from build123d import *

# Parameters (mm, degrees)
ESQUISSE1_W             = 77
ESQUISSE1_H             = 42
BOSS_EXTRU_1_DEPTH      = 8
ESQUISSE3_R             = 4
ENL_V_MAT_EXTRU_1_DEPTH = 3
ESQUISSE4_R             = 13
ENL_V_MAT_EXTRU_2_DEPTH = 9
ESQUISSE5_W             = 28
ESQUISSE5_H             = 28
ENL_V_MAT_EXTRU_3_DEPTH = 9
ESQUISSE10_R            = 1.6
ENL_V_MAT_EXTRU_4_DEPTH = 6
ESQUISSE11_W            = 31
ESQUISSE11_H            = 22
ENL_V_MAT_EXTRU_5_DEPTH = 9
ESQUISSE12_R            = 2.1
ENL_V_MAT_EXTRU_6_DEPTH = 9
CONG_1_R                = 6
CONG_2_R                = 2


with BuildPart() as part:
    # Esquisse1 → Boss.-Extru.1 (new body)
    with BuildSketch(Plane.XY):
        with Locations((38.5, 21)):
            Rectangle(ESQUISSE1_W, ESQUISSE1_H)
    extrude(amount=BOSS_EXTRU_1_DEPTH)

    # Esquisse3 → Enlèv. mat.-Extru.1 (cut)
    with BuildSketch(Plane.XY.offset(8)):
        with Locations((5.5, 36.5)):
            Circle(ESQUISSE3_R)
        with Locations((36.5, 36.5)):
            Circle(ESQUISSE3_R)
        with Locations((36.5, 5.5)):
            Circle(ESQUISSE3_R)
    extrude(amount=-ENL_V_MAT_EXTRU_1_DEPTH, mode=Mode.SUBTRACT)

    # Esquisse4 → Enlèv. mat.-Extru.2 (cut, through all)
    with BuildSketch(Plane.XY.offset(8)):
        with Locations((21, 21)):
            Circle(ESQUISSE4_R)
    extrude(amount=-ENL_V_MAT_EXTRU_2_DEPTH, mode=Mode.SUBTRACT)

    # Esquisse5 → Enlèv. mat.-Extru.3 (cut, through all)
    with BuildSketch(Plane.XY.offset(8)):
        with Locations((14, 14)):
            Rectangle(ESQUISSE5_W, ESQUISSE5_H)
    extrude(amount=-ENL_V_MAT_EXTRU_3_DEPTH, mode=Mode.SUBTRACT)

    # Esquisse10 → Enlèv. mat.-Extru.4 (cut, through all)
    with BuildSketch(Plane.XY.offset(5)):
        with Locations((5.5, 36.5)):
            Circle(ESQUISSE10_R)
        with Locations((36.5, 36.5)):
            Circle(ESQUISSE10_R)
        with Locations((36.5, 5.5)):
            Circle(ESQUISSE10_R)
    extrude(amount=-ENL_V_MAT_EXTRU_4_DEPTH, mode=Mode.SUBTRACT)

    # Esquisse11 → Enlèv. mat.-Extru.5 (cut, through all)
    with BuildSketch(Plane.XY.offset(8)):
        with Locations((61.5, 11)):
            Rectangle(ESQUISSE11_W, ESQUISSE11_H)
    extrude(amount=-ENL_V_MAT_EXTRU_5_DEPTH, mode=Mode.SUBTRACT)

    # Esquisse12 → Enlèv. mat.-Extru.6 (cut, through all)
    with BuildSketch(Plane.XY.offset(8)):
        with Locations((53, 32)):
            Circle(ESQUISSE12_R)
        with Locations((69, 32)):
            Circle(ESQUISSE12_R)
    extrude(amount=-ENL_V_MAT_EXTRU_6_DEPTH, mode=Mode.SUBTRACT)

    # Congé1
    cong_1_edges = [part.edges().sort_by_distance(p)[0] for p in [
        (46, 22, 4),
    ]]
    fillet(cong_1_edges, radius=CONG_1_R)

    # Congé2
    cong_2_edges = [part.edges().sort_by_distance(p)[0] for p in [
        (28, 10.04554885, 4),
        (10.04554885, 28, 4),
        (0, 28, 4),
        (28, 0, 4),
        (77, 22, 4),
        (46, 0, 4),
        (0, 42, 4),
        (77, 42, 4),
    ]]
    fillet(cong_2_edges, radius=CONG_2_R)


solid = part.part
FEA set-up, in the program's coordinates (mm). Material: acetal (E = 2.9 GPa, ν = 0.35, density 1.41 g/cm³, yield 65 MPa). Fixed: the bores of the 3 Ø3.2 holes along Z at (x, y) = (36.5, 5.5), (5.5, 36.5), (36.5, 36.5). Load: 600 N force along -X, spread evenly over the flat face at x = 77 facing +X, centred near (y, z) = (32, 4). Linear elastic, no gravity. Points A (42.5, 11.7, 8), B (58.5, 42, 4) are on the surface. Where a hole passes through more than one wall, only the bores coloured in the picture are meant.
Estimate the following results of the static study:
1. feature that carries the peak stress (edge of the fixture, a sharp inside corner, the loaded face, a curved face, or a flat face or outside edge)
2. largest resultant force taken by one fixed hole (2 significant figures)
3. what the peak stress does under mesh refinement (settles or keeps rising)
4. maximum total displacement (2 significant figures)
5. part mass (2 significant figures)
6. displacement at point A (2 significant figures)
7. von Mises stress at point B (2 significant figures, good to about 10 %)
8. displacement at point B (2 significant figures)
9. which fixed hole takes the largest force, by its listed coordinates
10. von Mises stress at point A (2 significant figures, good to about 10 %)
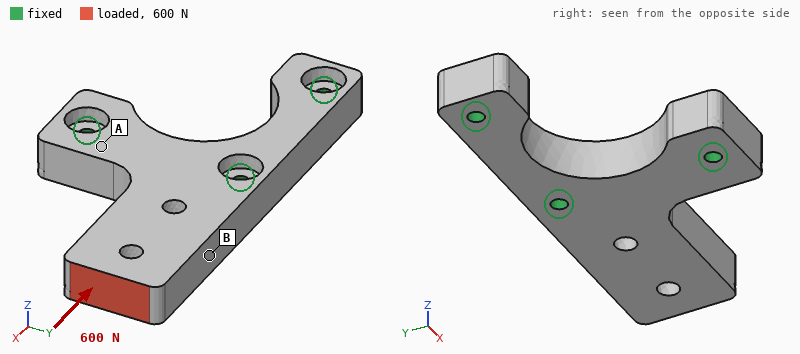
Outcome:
edge of the fixture
470 N
keeps rising
0.16 mm
17 g
0.025 mm
4.4 MPa
0.080 mm
(36.5, 36.5)
1.8 MPa
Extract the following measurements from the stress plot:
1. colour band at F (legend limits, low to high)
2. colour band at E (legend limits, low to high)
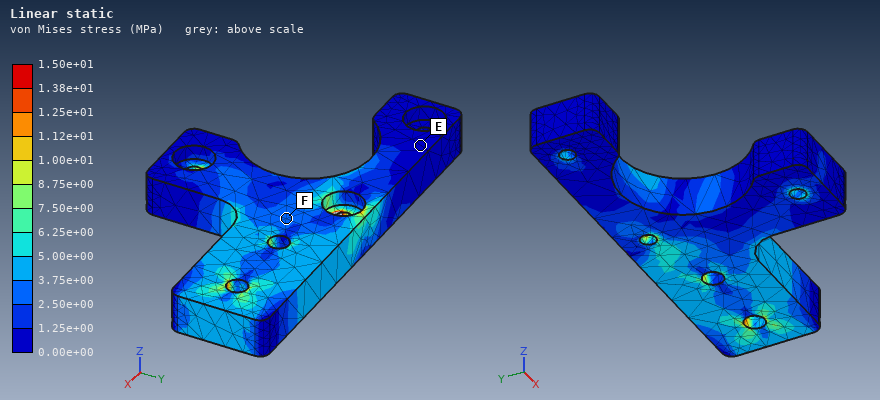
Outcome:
2.50e+00 to 3.75e+00 MPa
0.00e+00 to 1.25e+00 MPa
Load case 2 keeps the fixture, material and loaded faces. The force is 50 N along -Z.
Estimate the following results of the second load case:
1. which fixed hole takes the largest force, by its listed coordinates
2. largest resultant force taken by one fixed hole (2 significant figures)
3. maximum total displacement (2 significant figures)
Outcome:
(36.5, 36.5)
74 N
0.67 mm
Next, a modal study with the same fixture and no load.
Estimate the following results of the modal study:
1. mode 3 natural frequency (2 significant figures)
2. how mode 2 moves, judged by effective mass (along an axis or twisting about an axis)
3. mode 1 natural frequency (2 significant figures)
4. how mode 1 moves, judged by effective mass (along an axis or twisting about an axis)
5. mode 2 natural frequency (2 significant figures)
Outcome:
3500 Hz
along Y
900 Hz
along Z
2400 Hz
